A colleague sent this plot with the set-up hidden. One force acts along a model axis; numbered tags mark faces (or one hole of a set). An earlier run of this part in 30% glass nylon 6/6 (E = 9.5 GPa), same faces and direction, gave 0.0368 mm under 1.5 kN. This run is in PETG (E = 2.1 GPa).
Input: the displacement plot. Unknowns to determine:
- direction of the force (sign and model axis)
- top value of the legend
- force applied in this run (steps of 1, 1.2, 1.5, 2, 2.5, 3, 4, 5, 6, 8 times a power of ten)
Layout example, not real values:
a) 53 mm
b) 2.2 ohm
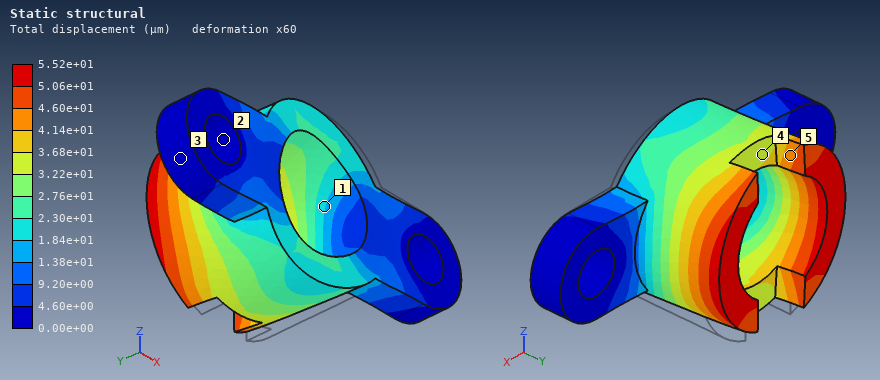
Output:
a) -X
b) 5.52e+01 µm
c) 500 N
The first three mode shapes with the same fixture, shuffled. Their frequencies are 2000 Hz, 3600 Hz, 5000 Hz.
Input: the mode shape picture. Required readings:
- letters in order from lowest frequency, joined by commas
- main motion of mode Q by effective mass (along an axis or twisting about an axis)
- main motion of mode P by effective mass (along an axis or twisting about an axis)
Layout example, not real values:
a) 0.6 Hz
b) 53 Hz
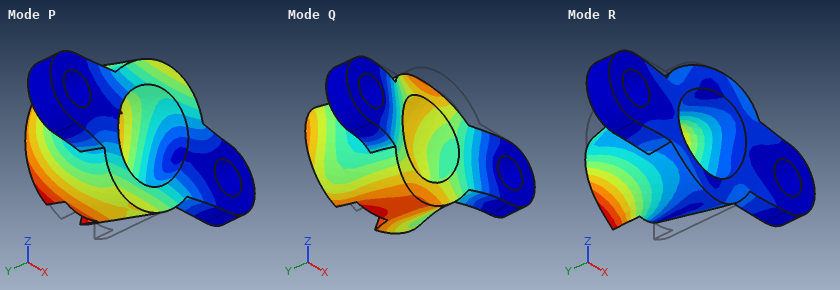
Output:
a) P, Q, R
b) along Y
c) along Z
